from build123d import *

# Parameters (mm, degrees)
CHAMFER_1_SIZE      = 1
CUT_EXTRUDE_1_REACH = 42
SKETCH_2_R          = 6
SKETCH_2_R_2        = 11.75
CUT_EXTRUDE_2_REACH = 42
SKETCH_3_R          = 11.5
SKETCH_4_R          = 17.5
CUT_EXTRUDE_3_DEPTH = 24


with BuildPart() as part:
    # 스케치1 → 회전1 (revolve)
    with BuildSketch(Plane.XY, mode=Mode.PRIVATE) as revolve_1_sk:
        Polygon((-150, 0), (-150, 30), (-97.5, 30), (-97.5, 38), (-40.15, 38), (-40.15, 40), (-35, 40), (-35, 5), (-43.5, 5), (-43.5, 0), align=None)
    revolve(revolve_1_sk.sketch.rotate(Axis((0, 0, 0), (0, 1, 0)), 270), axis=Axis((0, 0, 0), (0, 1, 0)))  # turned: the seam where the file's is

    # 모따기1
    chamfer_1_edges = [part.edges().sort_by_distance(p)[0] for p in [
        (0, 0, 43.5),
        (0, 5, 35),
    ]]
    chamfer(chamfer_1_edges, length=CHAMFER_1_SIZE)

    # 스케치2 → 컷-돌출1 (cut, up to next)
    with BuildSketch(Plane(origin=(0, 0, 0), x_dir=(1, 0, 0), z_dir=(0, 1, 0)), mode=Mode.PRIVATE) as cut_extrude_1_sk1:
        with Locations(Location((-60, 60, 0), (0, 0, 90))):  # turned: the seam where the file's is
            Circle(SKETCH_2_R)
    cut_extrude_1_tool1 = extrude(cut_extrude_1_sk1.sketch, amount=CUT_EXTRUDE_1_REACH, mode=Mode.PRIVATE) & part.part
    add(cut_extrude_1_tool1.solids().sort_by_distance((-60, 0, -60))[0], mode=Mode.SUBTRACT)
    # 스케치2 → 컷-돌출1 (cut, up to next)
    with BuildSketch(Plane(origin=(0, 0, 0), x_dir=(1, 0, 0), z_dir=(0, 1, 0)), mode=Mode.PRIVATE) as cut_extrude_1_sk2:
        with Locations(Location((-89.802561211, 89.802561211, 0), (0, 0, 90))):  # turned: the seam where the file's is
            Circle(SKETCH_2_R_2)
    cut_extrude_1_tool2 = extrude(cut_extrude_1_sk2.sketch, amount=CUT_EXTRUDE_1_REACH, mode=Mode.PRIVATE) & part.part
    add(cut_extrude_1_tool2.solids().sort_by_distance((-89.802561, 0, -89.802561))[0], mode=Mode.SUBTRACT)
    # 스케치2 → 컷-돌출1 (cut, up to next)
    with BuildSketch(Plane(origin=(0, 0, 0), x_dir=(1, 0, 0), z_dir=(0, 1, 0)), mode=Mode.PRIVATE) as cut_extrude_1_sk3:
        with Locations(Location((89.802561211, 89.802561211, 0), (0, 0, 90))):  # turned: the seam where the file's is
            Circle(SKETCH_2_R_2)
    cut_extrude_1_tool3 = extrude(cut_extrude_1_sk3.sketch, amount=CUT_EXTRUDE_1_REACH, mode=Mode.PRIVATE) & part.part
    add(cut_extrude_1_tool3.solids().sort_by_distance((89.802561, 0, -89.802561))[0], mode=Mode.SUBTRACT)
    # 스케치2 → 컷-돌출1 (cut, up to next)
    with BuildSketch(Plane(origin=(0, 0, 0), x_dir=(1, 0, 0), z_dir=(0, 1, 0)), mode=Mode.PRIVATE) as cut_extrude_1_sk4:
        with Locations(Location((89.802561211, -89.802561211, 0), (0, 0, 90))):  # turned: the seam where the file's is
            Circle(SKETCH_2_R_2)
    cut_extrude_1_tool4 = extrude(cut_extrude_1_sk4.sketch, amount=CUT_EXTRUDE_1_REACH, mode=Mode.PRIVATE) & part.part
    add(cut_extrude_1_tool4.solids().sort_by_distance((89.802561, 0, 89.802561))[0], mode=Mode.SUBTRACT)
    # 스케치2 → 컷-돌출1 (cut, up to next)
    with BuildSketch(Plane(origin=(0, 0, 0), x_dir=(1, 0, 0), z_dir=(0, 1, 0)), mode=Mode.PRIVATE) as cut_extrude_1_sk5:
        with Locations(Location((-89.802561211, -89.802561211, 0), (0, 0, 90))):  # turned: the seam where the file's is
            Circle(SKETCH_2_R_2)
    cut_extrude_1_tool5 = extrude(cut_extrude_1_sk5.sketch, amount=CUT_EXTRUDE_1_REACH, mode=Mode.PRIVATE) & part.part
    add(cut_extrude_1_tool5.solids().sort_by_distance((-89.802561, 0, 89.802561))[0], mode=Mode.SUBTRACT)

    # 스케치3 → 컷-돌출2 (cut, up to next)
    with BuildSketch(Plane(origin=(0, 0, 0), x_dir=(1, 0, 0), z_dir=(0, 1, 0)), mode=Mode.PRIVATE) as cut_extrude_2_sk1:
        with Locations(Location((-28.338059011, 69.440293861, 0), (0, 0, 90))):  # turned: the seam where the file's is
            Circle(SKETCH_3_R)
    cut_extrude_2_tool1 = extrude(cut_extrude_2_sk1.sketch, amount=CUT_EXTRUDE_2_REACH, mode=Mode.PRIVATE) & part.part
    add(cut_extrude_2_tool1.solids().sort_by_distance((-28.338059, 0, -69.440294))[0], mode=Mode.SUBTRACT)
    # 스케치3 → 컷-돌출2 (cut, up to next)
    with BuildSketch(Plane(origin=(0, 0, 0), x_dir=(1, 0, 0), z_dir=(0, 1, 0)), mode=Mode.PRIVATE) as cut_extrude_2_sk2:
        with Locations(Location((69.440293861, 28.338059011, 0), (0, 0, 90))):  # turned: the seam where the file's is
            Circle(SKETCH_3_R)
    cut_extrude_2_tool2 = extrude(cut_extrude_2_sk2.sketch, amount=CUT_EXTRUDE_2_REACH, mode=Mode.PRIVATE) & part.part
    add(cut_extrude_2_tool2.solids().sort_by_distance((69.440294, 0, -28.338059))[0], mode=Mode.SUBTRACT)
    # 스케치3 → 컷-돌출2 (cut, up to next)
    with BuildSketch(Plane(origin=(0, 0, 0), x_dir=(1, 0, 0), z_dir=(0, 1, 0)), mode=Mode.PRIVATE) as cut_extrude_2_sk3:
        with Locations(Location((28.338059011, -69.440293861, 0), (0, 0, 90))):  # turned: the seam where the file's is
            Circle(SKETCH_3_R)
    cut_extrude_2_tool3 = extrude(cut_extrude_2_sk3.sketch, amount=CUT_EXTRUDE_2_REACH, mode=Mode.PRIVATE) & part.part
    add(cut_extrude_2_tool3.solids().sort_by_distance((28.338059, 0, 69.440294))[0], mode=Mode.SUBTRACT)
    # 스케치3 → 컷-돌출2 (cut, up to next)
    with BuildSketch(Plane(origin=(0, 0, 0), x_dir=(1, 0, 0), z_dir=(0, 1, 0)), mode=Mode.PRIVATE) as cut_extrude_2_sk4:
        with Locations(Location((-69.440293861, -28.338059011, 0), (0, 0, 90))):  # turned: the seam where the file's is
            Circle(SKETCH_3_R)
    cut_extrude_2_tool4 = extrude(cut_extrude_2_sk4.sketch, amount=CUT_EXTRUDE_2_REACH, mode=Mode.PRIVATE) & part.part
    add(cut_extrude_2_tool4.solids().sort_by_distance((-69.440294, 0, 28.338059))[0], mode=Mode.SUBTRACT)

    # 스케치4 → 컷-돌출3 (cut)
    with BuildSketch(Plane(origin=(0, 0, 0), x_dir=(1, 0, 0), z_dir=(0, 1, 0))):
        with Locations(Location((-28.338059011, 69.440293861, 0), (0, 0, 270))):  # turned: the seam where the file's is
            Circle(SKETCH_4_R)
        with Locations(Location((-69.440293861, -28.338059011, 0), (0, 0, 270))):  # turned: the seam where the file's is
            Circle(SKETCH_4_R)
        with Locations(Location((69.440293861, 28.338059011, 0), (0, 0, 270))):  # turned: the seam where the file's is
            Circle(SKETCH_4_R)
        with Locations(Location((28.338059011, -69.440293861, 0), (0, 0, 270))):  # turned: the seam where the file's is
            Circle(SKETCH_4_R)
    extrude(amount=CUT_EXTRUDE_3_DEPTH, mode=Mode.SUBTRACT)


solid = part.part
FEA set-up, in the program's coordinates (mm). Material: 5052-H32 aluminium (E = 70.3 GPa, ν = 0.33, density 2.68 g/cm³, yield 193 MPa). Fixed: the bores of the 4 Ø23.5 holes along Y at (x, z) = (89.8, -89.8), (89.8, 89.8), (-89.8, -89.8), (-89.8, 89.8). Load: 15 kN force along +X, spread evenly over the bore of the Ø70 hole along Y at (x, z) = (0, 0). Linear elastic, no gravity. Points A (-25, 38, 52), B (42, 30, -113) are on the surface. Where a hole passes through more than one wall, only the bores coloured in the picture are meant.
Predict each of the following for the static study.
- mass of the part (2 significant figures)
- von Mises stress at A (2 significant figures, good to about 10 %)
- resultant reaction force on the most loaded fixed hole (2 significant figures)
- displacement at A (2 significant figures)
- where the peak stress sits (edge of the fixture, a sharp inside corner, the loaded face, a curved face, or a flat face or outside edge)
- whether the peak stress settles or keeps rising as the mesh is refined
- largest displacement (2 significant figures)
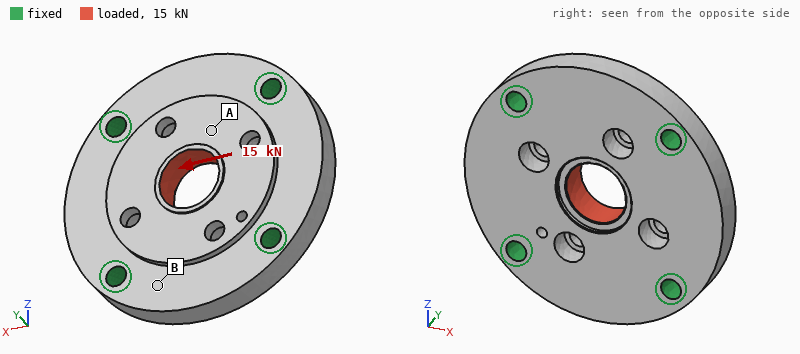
5.4 kg
1.7 MPa
4.2 kN
2.3 µm
edge of the fixture
keeps rising
4.8 µm
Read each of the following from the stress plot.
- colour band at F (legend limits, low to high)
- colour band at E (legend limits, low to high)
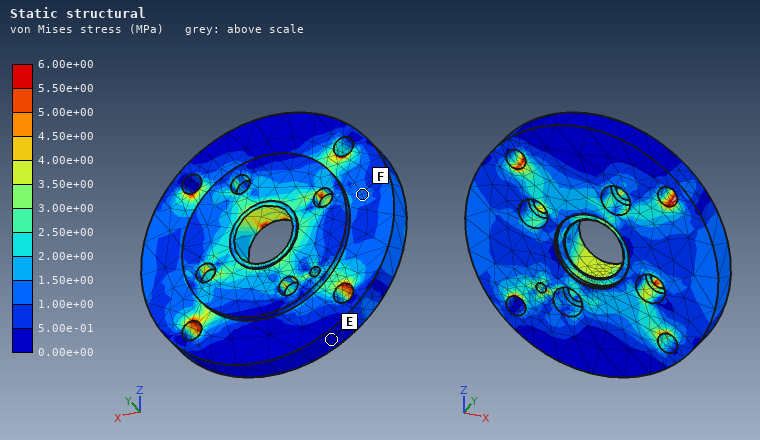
1.00e+00 to 1.50e+00 MPa
0.00e+00 to 5.00e-01 MPa
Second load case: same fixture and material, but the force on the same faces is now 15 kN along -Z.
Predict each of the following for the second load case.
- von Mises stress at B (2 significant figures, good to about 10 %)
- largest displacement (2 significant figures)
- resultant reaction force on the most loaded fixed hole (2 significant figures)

1.1 MPa
4.9 µm
4.1 kN
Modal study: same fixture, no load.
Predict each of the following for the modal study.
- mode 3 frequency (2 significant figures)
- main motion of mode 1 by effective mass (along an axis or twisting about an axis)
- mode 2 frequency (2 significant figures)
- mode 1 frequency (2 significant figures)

3900 Hz
along Y
3700 Hz
3500 Hz
